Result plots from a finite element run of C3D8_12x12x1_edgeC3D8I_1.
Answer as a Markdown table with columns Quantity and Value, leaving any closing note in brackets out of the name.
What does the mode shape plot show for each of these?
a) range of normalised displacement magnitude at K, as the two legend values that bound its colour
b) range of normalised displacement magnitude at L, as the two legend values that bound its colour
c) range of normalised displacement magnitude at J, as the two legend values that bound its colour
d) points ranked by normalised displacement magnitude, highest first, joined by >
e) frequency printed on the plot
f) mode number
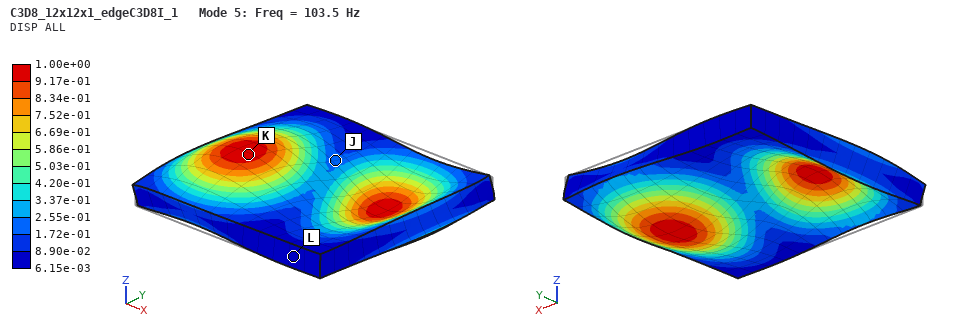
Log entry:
| Quantity | Value |
|---|---|
| range of normalised displacement magnitude at K, as the two legend values that bound its colour | 9.17e-01 to 1.00e+00 |
| range of normalised displacement magnitude at L, as the two legend values that bound its colour | 6.15e-03 to 8.90e-02 |
| range of normalised displacement magnitude at J, as the two legend values that bound its colour | 1.72e-01 to 2.55e-01 |
| points ranked by normalised displacement magnitude, highest first, joined by > | K > J > L |
| frequency printed on the plot | 103.5 Hz |
| mode number | 5 |
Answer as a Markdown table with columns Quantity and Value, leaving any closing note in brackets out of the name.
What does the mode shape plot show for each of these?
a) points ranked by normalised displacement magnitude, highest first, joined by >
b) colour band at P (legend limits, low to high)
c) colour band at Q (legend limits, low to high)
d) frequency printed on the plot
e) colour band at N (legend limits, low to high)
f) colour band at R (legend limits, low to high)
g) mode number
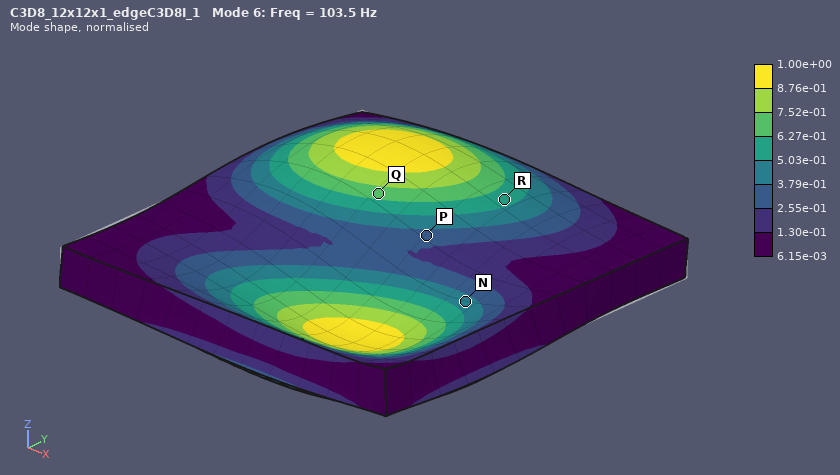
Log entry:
| Quantity | Value |
|---|---|
| points ranked by normalised displacement magnitude, highest first, joined by > | Q > R > N > P |
| colour band at P | 2.55e-01 to 3.79e-01 |
| colour band at Q | 6.27e-01 to 7.52e-01 |
| frequency printed on the plot | 103.5 Hz |
| colour band at N | 3.79e-01 to 5.03e-01 |
| colour band at R | 5.03e-01 to 6.27e-01 |
| mode number | 6 |
